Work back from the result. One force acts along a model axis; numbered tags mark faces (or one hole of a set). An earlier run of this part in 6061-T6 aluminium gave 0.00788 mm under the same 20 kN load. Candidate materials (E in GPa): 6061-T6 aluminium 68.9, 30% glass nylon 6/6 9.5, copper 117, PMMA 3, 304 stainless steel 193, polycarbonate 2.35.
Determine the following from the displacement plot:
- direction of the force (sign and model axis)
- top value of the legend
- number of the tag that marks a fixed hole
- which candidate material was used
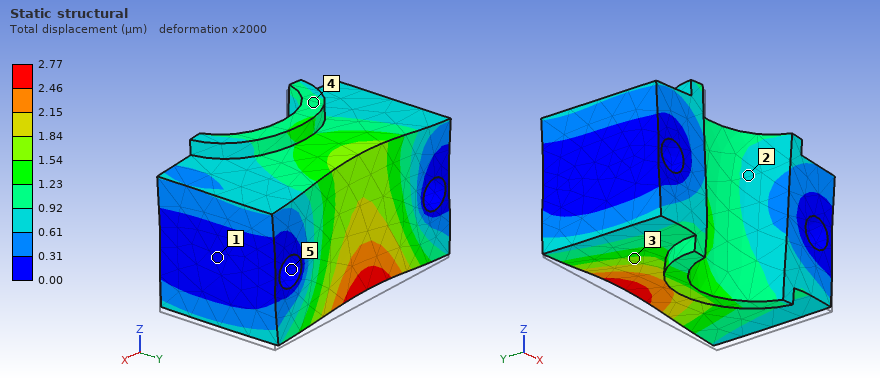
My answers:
+Z
2.77 µm
5
304 stainless steel
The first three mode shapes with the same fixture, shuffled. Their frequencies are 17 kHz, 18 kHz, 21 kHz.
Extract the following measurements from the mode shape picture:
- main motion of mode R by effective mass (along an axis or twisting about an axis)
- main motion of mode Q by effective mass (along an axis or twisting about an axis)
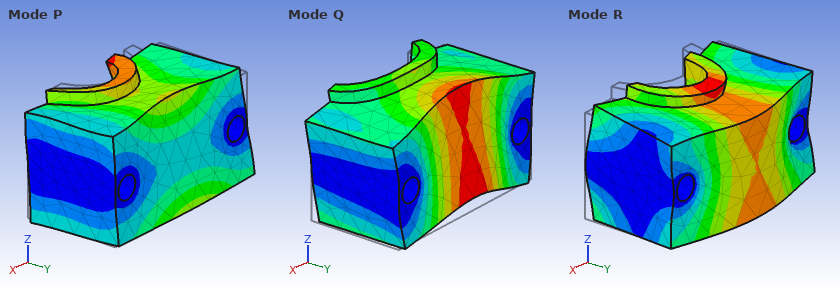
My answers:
along Y
along Z
